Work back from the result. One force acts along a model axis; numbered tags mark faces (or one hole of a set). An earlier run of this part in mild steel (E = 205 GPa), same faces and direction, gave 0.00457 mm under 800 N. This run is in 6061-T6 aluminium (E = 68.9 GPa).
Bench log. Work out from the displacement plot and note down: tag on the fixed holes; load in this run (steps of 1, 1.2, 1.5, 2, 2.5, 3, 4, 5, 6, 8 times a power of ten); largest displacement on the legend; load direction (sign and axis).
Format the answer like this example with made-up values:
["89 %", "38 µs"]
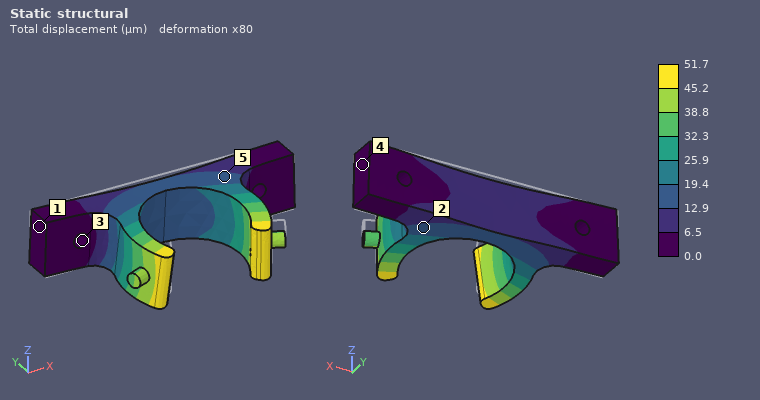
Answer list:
["3", "3 kN", "51.7 µm", "-Z"]
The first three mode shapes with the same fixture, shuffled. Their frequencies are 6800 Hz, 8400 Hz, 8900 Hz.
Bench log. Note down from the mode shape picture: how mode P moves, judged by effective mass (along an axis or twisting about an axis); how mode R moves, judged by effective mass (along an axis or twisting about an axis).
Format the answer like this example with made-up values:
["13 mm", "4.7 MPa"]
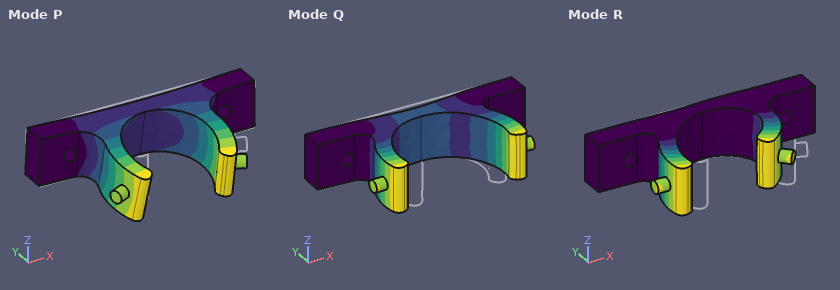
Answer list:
["along Z", "along X"]
